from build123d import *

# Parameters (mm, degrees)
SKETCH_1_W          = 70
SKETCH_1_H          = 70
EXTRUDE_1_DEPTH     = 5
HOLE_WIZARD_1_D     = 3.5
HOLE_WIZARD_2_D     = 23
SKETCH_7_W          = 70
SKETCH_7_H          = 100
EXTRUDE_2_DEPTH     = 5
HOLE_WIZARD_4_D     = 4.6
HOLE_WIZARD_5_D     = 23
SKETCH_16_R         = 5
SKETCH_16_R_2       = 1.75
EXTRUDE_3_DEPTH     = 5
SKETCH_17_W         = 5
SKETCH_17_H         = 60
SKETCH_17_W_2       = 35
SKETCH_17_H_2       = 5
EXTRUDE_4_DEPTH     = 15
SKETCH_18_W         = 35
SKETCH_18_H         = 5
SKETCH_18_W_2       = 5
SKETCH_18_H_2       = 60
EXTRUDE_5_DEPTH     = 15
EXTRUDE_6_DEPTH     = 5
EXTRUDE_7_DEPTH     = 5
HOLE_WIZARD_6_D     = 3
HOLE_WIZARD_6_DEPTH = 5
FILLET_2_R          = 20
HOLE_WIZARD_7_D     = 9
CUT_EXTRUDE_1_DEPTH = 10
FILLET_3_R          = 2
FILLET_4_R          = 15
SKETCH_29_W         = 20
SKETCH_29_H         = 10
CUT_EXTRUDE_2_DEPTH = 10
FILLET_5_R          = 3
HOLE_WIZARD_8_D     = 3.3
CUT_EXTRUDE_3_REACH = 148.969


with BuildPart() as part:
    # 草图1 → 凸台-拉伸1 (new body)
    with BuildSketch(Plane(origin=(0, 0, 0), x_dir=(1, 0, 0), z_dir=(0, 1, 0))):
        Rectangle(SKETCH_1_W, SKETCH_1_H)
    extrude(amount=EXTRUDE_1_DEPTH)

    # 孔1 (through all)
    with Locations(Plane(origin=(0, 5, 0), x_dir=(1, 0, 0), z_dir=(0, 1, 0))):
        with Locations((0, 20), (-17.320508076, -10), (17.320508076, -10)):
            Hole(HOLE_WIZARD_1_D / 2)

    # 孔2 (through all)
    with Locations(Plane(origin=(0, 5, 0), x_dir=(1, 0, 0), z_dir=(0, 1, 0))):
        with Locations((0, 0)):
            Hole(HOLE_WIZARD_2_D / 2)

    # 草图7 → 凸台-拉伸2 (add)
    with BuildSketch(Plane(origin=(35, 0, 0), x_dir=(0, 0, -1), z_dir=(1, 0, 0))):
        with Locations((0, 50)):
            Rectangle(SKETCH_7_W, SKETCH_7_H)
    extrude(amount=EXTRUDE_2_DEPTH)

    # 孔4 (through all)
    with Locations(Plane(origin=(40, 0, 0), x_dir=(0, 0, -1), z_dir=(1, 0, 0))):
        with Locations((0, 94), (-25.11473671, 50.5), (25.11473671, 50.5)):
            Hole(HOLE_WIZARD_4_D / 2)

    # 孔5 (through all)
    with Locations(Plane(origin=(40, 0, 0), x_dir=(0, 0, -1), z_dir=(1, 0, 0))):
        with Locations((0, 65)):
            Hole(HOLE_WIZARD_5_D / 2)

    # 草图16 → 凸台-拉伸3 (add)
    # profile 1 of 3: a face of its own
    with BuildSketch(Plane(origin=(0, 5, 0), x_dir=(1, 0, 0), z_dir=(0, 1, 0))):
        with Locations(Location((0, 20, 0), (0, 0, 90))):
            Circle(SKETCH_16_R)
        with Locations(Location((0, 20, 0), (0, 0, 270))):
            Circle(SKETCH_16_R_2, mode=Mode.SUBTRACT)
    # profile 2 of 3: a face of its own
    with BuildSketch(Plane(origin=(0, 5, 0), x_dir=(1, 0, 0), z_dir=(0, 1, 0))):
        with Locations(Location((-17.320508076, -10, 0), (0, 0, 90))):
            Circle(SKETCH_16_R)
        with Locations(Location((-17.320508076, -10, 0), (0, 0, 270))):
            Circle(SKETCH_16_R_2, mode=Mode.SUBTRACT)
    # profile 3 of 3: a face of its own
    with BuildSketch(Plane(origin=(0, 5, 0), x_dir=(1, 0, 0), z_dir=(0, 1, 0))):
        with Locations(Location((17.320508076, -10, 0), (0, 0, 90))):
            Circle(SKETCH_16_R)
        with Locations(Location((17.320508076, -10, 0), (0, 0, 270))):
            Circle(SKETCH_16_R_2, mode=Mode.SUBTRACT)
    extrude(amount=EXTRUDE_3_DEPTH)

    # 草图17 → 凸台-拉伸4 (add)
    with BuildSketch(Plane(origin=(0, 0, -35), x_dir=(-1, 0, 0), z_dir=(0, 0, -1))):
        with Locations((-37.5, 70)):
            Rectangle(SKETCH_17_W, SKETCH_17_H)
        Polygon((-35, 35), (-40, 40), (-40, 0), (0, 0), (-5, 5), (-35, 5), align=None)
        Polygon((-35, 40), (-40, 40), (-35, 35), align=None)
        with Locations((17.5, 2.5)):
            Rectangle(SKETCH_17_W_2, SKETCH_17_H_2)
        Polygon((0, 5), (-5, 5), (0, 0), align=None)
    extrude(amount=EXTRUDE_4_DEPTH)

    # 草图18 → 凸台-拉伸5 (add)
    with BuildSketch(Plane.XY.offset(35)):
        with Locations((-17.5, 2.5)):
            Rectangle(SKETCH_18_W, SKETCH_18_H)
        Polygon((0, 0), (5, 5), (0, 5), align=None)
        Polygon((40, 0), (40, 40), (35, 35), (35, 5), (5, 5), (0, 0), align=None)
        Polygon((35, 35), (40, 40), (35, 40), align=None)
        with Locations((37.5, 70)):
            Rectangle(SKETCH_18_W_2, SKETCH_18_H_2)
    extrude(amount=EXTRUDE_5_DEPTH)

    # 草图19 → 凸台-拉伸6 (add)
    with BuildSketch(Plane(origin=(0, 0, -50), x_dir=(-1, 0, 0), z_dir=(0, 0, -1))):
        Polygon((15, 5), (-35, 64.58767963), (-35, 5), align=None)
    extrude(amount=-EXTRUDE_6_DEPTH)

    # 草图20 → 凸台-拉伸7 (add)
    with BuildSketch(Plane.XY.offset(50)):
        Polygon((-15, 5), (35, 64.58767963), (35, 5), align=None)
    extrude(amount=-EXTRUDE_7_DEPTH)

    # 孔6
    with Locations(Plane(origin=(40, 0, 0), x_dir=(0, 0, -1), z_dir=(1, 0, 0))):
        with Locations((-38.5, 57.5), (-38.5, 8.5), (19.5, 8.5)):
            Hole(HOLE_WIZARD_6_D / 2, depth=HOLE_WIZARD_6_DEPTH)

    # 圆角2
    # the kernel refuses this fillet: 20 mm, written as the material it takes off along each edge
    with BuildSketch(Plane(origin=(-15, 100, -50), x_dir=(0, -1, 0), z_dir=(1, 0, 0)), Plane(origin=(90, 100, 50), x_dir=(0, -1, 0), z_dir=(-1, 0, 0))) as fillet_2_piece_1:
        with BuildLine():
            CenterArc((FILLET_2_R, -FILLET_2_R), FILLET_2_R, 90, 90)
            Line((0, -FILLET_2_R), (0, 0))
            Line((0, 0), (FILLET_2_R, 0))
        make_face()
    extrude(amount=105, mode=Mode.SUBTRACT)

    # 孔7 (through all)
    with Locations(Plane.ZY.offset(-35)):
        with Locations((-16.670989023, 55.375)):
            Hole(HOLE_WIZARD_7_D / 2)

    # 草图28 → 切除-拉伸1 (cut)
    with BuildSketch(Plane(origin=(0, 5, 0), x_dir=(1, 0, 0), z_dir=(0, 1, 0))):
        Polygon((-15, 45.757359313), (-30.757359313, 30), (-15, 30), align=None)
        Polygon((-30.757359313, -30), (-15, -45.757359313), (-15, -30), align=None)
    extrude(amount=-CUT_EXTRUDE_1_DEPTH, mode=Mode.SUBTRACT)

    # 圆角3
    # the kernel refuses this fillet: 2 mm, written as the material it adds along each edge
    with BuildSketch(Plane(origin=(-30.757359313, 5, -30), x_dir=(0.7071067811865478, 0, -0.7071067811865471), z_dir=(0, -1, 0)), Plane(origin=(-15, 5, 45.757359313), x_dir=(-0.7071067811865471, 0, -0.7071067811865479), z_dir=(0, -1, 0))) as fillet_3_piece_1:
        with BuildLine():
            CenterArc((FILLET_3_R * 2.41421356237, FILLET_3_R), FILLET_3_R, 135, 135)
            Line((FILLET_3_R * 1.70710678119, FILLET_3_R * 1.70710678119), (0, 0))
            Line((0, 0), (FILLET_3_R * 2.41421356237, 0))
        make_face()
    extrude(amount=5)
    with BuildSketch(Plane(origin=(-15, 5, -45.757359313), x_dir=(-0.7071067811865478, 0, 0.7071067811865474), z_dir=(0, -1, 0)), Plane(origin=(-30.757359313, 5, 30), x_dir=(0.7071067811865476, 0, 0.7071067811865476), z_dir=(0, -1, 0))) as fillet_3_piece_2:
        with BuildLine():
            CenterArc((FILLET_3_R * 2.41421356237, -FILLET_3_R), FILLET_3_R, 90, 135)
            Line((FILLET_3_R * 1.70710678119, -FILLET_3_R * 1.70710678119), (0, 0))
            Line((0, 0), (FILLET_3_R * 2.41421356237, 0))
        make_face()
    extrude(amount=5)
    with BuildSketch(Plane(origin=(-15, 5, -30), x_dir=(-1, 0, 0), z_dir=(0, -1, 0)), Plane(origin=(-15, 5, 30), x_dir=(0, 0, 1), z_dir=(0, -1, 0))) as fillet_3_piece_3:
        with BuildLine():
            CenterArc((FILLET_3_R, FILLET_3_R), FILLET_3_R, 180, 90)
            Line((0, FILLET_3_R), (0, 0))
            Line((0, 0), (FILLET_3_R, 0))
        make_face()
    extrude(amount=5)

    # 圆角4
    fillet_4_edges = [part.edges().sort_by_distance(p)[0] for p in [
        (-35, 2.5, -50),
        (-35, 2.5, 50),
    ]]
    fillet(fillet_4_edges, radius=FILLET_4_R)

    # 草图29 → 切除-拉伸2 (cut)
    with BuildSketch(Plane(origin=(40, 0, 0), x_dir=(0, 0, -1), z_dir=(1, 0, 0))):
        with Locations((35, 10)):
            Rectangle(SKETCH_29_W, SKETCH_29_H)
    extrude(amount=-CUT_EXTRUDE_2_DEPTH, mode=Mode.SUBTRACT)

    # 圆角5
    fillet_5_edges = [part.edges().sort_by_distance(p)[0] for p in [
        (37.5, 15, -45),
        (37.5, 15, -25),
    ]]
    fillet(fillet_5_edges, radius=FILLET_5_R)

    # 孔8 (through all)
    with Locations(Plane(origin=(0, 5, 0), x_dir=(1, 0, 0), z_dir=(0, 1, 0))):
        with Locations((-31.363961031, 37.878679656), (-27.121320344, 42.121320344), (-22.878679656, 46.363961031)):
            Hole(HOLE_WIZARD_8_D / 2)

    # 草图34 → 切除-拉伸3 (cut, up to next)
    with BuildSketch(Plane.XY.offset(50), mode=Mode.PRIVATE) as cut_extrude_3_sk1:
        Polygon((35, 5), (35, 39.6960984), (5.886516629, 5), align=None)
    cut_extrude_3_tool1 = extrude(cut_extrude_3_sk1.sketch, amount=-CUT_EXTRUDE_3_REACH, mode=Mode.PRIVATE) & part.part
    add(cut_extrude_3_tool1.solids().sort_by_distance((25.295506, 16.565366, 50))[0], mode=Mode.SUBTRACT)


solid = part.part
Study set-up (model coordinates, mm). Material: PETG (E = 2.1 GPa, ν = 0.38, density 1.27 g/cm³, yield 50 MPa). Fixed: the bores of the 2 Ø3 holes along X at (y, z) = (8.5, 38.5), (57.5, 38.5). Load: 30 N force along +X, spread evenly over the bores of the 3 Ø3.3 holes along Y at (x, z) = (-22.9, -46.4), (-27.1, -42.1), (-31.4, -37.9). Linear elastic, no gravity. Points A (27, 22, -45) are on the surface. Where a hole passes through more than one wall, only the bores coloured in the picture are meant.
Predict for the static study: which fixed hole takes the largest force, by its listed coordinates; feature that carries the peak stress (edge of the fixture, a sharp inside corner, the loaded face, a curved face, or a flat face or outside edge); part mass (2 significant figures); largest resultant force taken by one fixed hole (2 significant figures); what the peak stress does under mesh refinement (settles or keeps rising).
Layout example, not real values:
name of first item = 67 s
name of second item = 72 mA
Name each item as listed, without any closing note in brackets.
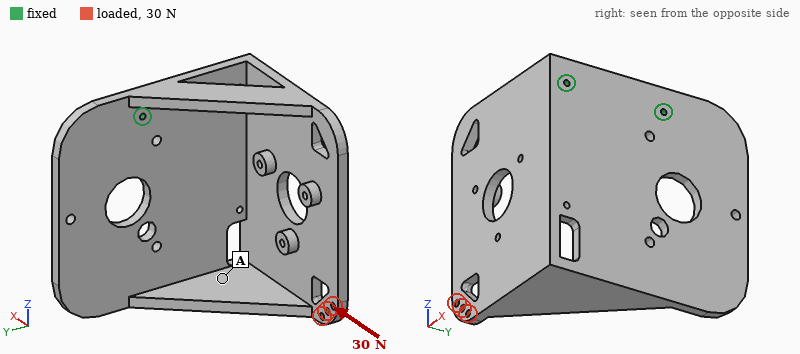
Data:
which fixed hole takes the largest force, by its listed coordinates = (8.5, 38.5)
feature that carries the peak stress = edge of the fixture
part mass = 110 g
largest resultant force taken by one fixed hole = 34 N
what the peak stress does under mesh refinement = keeps rising
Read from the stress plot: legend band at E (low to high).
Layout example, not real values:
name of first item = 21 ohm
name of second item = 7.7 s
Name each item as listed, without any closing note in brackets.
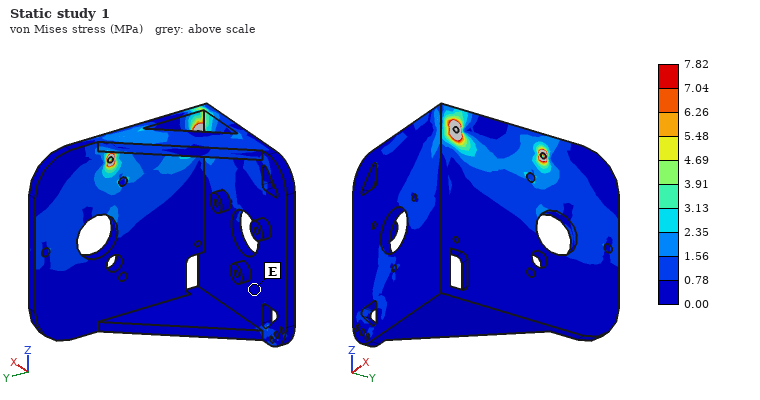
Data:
legend band at E = 0.00 to 0.78 MPa
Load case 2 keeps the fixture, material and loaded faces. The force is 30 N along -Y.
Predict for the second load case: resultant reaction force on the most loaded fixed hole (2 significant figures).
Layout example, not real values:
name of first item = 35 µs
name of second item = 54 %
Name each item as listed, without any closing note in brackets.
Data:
resultant reaction force on the most loaded fixed hole = 64 N
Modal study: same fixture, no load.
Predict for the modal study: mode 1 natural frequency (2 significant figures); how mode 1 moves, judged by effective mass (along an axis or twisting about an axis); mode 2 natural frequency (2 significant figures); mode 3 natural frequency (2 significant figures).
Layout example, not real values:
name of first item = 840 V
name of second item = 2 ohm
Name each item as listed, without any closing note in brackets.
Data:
mode 1 natural frequency = 100 Hz
how mode 1 moves, judged by effective mass = along X
mode 2 natural frequency = 170 Hz
mode 3 natural frequency = 390 Hz
